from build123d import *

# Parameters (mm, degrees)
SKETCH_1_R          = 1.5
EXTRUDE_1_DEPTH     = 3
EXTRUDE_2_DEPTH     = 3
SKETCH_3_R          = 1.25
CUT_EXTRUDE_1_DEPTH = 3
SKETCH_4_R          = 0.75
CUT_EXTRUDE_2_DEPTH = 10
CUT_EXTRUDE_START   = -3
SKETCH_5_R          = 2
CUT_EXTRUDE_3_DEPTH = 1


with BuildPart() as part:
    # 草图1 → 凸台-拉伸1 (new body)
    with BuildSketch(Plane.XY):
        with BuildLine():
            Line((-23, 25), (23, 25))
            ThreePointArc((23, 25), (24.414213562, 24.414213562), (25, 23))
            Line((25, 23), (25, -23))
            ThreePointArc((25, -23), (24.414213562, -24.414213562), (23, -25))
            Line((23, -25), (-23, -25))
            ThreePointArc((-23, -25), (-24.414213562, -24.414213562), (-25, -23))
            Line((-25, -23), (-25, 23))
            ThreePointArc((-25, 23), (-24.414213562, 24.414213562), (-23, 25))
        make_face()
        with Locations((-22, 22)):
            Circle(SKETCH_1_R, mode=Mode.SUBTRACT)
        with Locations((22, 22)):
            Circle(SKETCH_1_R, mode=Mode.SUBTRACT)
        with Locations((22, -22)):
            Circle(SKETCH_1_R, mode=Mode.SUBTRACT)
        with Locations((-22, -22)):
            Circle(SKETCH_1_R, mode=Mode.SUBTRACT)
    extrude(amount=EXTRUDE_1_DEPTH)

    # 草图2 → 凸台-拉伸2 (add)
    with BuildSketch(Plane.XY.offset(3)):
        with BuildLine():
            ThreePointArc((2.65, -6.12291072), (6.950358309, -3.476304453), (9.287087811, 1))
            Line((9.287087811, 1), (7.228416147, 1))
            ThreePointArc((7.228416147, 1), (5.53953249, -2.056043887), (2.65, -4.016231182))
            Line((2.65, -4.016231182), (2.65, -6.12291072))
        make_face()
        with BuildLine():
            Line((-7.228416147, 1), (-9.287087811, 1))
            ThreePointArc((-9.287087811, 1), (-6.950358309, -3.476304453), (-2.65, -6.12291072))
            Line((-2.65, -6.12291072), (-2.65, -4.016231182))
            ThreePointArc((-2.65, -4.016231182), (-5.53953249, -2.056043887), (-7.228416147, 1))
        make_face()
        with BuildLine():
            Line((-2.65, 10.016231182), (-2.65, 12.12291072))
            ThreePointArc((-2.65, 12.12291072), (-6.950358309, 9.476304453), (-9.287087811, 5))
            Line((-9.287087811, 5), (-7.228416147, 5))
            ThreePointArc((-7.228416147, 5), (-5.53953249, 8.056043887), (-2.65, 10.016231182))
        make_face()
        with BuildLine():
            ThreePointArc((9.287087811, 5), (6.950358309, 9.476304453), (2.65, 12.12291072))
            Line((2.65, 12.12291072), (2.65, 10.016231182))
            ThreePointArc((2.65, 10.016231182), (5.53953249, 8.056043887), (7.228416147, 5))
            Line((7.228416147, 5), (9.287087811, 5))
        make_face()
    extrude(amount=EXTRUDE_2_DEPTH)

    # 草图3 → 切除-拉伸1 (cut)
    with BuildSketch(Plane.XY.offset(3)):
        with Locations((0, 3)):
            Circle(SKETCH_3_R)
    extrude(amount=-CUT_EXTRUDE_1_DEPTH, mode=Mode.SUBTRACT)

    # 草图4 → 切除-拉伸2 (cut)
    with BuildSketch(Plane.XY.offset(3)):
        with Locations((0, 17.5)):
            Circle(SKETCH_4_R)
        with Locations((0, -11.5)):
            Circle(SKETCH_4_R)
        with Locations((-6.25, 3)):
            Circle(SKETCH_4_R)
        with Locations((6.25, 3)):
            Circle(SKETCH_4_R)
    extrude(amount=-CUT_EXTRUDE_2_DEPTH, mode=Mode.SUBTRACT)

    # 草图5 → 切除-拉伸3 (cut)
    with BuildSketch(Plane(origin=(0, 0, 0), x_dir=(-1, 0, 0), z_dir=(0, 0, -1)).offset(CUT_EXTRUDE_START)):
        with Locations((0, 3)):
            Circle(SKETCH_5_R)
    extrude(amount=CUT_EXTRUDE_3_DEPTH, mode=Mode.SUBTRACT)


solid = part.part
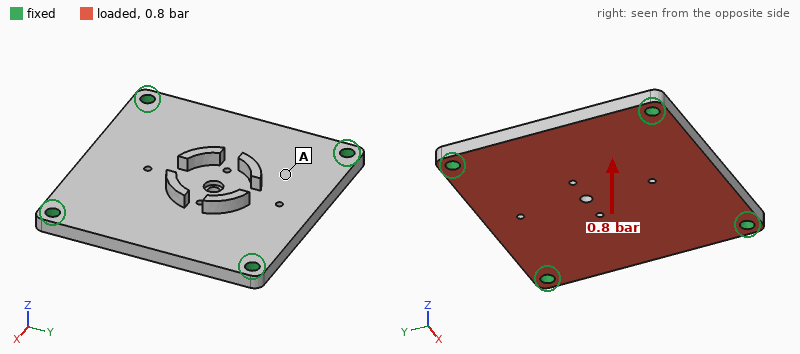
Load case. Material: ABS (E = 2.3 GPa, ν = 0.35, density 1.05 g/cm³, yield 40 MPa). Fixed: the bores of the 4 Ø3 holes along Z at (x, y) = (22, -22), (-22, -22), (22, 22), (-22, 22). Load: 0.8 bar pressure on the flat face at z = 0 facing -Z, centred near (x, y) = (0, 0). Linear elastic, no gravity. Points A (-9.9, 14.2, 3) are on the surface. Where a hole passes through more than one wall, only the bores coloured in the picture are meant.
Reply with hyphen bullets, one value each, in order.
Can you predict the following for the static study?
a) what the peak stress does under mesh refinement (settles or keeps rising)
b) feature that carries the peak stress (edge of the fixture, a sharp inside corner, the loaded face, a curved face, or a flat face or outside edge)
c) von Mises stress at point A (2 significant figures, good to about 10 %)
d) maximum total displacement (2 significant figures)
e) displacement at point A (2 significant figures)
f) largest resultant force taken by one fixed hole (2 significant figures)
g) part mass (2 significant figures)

- keeps rising
- edge of the fixture
- 3.2 MPa
- 0.41 mm
- 0.24 mm
- 49 N
- 7.9 g
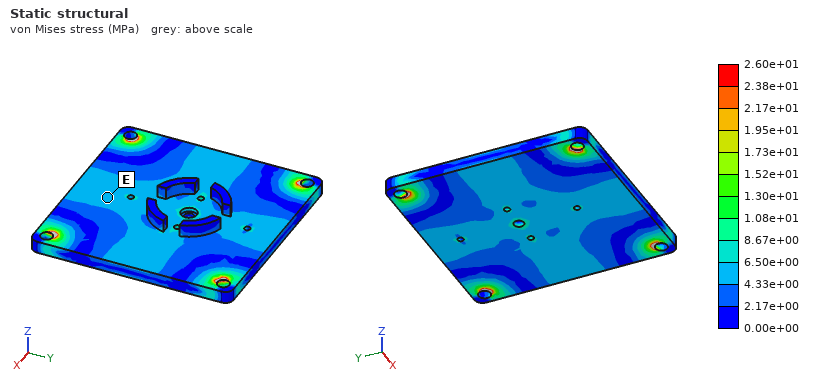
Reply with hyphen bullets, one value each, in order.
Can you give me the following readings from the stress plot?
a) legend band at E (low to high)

- 4.33e+00 to 6.50e+00 MPa
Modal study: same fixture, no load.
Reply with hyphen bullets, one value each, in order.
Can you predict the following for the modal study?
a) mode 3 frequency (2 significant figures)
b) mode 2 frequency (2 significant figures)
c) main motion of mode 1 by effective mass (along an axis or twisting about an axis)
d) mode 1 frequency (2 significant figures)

- 2600 Hz
- 2600 Hz
- along Z
- 1500 Hz
